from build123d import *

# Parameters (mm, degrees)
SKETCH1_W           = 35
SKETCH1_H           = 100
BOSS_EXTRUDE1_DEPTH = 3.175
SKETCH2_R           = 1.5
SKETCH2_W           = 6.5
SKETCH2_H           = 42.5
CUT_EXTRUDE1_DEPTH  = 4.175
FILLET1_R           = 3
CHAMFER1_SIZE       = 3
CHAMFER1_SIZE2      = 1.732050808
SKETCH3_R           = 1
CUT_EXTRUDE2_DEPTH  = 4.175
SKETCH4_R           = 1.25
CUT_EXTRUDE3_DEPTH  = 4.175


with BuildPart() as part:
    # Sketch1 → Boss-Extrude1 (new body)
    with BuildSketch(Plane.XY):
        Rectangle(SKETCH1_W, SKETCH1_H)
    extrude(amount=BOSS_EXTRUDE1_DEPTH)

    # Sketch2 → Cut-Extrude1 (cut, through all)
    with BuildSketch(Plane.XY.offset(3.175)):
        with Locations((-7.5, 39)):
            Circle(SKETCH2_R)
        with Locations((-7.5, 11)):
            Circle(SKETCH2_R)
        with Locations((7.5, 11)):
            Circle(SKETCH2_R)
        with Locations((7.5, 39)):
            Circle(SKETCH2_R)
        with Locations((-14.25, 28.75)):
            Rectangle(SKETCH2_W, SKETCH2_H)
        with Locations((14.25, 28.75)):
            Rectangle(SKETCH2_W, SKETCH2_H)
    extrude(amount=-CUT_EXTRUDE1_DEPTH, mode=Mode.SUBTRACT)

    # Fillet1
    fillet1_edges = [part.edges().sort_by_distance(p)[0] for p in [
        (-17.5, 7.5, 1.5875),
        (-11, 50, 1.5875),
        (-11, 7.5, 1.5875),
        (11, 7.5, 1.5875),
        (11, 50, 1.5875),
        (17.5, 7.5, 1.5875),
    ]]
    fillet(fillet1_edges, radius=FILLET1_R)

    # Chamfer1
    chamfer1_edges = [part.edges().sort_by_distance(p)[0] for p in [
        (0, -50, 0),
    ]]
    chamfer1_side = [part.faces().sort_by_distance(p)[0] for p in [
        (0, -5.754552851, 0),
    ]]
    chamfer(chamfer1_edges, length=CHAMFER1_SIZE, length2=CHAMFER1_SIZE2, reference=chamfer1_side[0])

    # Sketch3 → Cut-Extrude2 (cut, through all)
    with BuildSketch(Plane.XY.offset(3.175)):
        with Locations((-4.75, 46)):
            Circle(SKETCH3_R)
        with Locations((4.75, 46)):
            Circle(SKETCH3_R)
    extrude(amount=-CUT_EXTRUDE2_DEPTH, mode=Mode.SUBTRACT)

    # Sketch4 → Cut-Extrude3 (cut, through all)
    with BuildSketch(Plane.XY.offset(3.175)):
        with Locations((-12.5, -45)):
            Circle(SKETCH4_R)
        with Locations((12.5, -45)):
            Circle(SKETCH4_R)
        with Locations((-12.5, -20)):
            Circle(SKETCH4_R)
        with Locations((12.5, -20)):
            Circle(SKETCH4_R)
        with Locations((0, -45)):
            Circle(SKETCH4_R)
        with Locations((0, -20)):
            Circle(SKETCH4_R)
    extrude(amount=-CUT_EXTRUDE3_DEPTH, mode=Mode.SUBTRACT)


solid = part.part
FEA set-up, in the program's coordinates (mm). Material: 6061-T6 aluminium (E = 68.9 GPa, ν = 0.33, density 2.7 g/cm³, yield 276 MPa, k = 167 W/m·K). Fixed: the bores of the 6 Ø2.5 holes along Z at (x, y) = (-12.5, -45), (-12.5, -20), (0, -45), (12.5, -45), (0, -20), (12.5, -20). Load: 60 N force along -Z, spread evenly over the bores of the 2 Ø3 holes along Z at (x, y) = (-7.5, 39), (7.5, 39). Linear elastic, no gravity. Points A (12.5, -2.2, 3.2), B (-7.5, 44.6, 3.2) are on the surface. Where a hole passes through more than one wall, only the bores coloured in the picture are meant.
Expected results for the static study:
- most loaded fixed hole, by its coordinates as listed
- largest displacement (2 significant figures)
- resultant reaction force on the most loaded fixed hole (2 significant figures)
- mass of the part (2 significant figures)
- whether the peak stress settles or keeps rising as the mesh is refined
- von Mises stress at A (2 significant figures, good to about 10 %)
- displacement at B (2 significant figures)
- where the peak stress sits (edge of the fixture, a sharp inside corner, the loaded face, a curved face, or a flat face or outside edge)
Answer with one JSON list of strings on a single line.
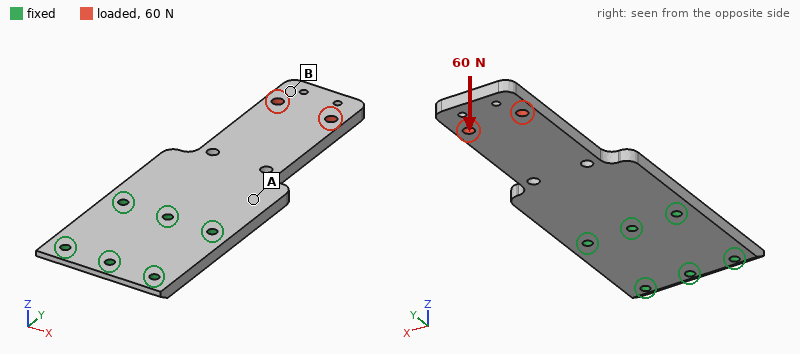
["(0, -20)", "0.94 mm", "80 N", "24 g", "keeps rising", "40 MPa", "0.83 mm", "edge of the fixture"]
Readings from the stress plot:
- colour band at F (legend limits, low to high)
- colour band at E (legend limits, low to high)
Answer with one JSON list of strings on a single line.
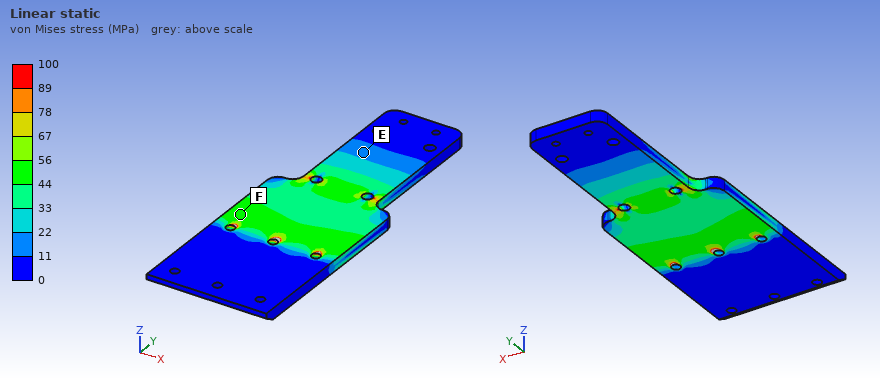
["44 to 56 MPa", "11 to 22 MPa"]
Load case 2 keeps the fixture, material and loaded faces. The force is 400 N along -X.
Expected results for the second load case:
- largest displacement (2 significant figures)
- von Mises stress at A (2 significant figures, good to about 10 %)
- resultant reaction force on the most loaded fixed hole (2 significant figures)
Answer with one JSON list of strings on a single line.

["98 µm", "22 MPa", "820 N"]
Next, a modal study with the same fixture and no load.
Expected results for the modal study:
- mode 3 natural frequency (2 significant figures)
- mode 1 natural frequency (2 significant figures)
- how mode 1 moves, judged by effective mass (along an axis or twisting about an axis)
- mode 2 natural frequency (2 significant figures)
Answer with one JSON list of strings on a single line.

["3700 Hz", "650 Hz", "along Z", "3400 Hz"]
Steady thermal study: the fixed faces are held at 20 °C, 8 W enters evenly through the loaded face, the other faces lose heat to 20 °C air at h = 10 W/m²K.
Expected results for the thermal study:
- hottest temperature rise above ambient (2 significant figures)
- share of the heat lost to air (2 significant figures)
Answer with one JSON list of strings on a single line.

["35 K", "8.7 %"]
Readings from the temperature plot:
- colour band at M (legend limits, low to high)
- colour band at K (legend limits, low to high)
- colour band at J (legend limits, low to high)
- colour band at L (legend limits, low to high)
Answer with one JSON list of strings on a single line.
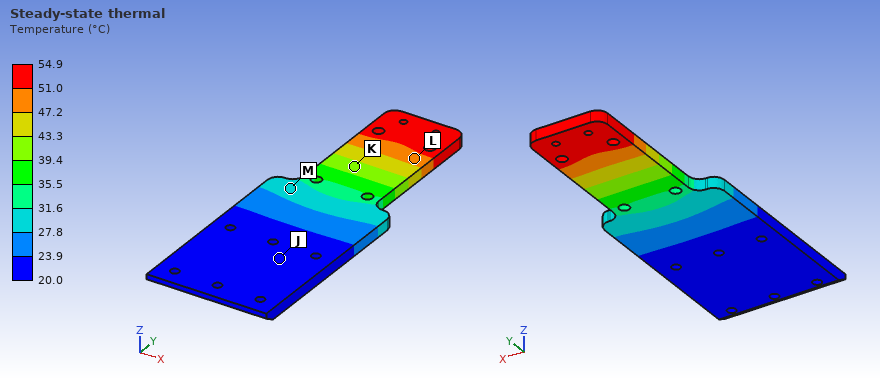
["27.8 to 31.6 °C", "39.4 to 43.3 °C", "20.0 to 23.9 °C", "47.2 to 51.0 °C"]
